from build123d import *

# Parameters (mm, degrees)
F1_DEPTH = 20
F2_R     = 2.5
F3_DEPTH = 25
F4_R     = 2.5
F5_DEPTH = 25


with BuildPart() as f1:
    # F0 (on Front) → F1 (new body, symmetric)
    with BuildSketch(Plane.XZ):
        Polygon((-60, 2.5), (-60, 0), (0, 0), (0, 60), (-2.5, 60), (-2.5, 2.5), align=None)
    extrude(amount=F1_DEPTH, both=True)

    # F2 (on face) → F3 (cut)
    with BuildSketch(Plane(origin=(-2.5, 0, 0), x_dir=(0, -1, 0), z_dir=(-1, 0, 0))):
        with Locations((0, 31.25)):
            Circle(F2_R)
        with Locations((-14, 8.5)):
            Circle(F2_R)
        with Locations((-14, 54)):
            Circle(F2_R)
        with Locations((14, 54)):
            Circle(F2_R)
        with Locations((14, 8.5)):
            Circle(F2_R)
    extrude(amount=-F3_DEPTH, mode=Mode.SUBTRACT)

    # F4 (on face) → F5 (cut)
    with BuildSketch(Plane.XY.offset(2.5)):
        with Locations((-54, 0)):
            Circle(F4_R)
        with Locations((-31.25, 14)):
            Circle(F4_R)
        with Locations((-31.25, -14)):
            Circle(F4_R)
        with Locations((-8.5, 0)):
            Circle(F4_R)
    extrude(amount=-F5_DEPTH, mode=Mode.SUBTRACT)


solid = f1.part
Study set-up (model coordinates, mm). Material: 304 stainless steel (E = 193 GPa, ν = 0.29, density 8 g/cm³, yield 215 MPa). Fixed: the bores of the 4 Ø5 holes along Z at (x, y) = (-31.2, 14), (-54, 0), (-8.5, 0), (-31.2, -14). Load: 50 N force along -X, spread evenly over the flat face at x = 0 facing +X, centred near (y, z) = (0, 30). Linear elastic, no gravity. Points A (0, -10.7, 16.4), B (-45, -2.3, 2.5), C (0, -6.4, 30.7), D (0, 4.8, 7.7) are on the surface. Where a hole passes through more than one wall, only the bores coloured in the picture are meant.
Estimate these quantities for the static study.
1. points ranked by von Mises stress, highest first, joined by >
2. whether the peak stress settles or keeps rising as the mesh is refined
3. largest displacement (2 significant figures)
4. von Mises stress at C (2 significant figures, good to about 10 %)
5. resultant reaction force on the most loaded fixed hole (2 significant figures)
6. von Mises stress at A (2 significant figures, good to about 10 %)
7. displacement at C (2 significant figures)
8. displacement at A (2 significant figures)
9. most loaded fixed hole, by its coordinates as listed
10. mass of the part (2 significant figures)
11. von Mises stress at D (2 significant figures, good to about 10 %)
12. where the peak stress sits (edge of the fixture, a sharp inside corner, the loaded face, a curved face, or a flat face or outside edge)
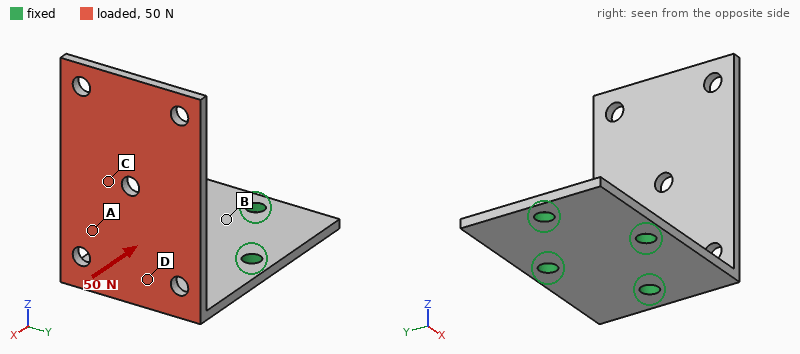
D > A > C > B
keeps rising
0.19 mm
9.7 MPa
44 N
17 MPa
0.075 mm
0.030 mm
(-8.5, 0)
90 g
30 MPa
edge of the fixture
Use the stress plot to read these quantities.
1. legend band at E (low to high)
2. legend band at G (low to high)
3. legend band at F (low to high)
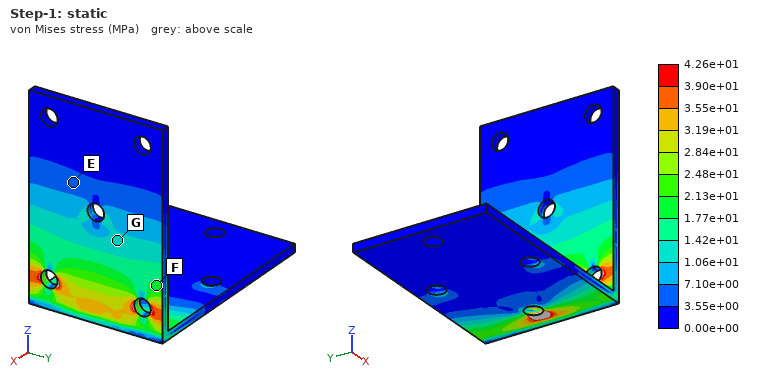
3.55e+00 to 7.10e+00 MPa
1.06e+01 to 1.42e+01 MPa
1.77e+01 to 2.13e+01 MPa
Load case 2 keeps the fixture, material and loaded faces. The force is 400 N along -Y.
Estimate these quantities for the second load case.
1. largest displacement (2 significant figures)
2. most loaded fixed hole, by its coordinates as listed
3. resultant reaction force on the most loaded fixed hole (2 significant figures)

0.28 mm
(-8.5, 0)
410 N
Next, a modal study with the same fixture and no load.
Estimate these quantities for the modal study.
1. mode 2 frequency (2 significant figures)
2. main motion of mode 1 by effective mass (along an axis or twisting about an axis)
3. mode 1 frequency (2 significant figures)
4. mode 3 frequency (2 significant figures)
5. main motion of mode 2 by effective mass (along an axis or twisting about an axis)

1000 Hz
along X
480 Hz
1800 Hz
along Y
